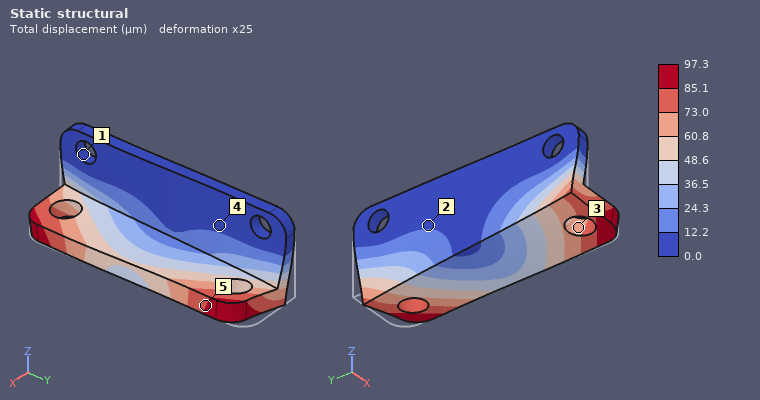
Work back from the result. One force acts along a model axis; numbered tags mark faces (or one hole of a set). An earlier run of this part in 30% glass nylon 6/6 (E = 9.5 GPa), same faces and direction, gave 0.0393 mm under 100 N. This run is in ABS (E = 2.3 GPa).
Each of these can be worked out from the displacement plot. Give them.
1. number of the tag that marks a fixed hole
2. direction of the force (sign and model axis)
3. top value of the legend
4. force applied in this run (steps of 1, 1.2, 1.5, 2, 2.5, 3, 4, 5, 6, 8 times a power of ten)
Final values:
1
-Y
97.3 µm
60 N
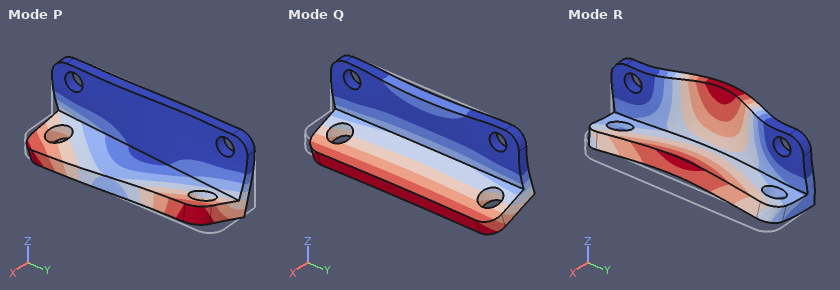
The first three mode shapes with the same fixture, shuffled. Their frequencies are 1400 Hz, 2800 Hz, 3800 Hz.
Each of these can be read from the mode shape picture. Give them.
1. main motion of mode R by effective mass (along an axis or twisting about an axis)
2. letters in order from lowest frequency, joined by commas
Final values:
along X
Q, P, R
